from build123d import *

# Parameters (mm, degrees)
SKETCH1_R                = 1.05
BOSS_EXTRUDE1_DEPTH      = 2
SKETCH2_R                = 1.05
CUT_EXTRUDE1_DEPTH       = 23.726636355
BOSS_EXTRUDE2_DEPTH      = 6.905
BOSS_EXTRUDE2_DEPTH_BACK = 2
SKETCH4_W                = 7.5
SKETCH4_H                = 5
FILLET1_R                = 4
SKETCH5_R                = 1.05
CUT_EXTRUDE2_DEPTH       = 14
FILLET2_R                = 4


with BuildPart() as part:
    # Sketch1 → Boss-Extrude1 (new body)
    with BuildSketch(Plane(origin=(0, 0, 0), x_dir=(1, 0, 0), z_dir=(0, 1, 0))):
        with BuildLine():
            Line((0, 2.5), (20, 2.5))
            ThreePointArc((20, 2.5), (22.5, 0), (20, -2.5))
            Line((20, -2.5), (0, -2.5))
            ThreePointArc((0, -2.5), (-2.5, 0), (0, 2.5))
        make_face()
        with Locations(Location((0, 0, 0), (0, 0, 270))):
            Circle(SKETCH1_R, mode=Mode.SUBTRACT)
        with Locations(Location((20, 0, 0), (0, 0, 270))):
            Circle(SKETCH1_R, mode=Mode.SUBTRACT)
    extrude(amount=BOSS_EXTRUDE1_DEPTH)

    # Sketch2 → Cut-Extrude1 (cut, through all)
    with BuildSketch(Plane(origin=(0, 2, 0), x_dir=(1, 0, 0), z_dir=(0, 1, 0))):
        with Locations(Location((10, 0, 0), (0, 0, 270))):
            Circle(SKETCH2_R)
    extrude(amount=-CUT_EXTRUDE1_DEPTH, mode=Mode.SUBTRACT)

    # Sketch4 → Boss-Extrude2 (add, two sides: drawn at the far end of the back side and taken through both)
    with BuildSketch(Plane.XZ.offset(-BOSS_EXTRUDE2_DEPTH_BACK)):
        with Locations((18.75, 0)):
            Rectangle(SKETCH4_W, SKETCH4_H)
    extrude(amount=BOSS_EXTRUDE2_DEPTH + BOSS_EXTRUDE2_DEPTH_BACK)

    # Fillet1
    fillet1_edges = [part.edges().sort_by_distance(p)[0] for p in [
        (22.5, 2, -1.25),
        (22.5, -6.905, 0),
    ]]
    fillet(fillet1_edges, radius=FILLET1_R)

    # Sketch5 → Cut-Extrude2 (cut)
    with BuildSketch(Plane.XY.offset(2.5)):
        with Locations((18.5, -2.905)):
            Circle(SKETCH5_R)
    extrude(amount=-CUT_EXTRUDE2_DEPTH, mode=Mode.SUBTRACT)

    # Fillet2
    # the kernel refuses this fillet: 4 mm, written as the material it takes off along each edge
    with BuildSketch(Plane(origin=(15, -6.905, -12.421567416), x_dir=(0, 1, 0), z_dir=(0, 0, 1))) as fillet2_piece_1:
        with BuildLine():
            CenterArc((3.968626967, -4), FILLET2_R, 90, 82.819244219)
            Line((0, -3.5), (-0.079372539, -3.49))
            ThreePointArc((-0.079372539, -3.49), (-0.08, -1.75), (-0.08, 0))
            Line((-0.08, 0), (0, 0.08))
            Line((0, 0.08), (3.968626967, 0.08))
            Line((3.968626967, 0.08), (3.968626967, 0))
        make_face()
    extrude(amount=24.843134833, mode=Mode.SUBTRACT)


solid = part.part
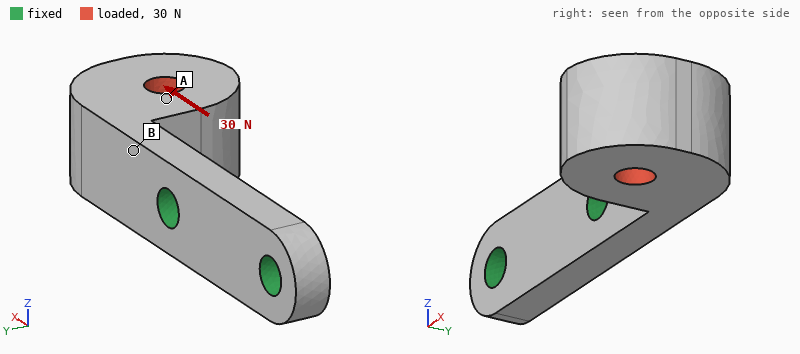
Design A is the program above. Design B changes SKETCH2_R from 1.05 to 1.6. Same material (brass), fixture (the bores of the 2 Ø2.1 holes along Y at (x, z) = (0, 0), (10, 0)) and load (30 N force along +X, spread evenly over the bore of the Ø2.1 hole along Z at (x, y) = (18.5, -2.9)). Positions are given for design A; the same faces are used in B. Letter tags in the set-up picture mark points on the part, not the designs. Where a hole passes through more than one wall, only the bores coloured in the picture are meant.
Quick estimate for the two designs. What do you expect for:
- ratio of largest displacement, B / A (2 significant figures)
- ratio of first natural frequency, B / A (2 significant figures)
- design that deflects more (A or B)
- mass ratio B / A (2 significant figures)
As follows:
0.85
1.1
A
0.98
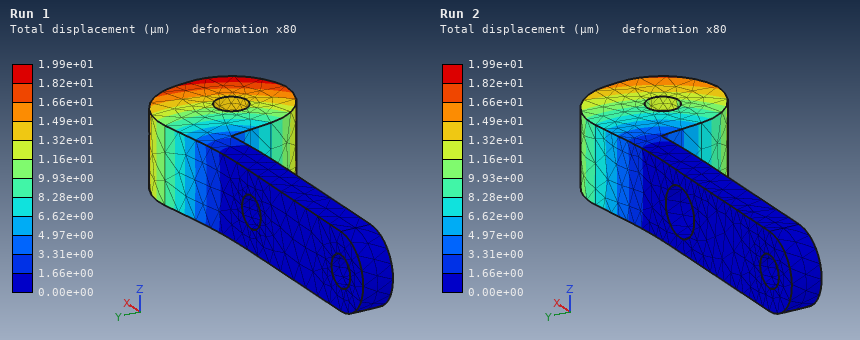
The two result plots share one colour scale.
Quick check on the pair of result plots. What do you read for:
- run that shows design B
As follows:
Run 2
